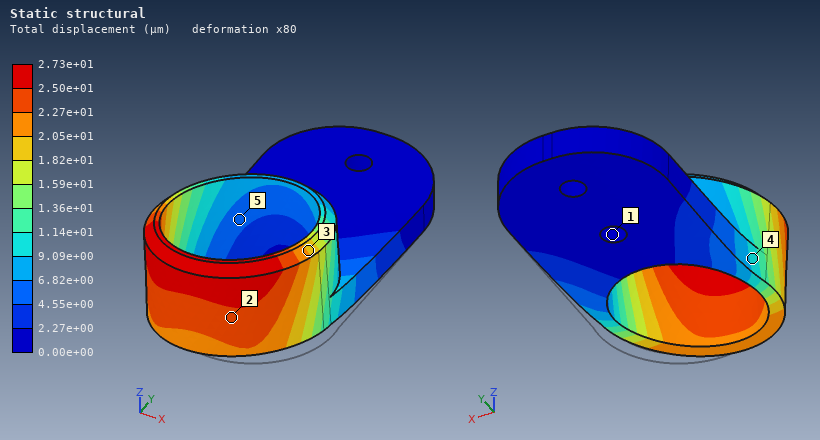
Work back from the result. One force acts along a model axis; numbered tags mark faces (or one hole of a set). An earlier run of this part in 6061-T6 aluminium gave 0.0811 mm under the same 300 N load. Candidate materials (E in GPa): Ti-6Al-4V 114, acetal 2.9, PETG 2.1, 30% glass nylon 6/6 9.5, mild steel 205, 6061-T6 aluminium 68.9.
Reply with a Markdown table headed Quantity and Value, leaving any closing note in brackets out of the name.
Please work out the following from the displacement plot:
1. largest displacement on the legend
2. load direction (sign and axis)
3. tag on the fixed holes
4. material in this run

| Quantity | Value |
|---|---|
| largest displacement on the legend | 2.73e+01 µm |
| load direction | -X |
| tag on the fixed holes | 1 |
| material in this run | mild steel |
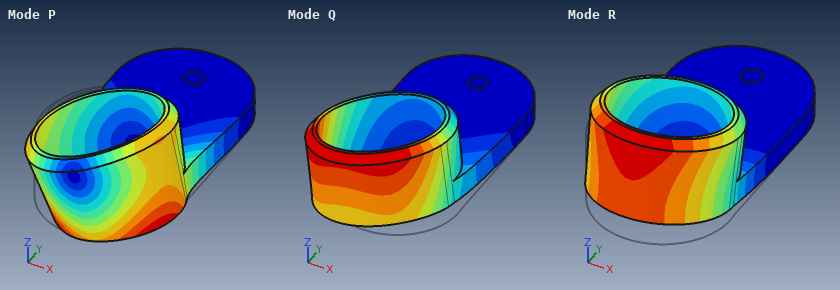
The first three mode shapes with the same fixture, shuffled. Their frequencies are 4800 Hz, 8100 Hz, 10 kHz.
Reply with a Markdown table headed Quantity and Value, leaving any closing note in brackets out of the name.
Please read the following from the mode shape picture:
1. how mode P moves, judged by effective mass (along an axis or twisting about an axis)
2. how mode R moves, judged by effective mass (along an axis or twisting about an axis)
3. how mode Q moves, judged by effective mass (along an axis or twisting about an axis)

| Quantity | Value |
|---|---|
| how mode P moves, judged by effective mass | twisting about Y |
| how mode R moves, judged by effective mass | along Z |
| how mode Q moves, judged by effective mass | along X |
